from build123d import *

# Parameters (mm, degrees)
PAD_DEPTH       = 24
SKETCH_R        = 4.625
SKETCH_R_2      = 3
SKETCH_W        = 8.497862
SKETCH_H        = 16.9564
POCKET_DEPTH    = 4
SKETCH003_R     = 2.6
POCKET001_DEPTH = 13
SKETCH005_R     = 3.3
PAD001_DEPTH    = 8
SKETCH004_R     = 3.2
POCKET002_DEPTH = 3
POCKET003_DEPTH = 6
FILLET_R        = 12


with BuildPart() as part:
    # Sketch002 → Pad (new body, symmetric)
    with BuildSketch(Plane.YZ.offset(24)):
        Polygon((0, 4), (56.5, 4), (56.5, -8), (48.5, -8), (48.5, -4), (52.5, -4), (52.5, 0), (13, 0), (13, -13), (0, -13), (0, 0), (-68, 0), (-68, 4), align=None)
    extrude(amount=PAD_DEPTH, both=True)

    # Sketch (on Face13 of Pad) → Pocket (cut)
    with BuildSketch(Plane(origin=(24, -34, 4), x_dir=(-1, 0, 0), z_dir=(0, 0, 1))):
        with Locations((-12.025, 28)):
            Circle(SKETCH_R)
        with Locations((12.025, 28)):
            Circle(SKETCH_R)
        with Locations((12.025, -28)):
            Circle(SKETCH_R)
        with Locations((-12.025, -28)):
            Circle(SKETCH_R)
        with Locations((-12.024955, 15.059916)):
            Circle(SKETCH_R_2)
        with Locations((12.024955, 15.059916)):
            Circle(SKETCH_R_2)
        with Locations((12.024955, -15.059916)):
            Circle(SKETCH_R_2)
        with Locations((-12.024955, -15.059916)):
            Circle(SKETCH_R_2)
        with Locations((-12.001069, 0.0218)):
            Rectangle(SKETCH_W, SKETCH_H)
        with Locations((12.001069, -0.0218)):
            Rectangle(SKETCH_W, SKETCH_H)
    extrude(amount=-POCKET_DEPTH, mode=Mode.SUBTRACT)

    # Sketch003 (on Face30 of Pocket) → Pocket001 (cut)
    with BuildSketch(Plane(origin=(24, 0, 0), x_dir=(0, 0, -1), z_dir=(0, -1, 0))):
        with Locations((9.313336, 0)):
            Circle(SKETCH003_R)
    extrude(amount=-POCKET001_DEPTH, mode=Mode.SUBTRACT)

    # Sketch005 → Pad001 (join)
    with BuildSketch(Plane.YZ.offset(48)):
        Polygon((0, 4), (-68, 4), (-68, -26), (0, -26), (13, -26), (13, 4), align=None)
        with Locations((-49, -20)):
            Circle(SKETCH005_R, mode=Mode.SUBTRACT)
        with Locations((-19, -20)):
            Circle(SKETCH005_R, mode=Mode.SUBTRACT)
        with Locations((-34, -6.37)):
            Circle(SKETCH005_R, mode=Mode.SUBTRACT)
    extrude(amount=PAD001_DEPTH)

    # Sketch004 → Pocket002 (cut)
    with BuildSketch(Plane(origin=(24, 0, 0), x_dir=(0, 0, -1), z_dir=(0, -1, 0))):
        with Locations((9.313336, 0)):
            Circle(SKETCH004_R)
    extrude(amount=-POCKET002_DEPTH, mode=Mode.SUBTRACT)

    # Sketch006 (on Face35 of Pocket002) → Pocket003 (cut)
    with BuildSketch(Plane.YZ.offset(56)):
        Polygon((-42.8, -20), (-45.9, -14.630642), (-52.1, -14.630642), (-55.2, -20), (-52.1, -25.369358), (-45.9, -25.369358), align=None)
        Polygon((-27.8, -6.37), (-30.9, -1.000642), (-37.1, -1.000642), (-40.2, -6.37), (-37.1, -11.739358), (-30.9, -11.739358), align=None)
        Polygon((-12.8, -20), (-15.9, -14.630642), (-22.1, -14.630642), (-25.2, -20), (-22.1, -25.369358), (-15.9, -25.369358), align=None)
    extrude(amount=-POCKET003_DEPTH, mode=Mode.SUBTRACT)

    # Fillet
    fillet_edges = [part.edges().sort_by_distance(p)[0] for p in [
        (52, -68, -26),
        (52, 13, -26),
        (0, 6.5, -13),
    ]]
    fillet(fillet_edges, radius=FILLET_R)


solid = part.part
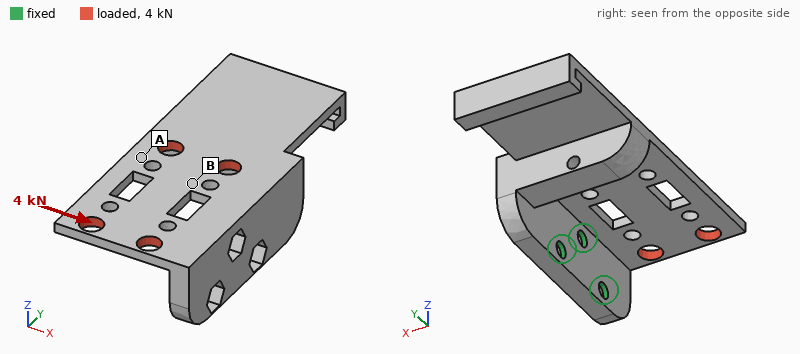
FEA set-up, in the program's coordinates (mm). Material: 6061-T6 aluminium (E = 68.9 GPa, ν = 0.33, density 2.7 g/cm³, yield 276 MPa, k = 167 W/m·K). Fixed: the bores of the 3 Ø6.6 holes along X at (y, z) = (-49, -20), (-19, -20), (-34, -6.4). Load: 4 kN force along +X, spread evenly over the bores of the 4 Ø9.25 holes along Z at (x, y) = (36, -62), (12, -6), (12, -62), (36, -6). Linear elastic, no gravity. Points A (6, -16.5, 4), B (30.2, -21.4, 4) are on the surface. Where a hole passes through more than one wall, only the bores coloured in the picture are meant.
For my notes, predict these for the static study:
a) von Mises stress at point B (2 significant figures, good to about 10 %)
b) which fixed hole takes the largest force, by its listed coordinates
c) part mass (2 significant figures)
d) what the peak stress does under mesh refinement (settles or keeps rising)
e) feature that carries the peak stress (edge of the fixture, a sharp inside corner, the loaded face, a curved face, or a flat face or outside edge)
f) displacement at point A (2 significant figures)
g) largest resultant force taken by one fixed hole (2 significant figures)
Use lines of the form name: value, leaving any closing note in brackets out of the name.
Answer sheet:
von Mises stress at point B: 38 MPa
which fixed hole takes the largest force, by its listed coordinates: (-34, -6.4)
part mass: 130 g
what the peak stress does under mesh refinement: keeps rising
feature that carries the peak stress: edge of the fixture
displacement at point A: 0.19 mm
largest resultant force taken by one fixed hole: 5.0 kN
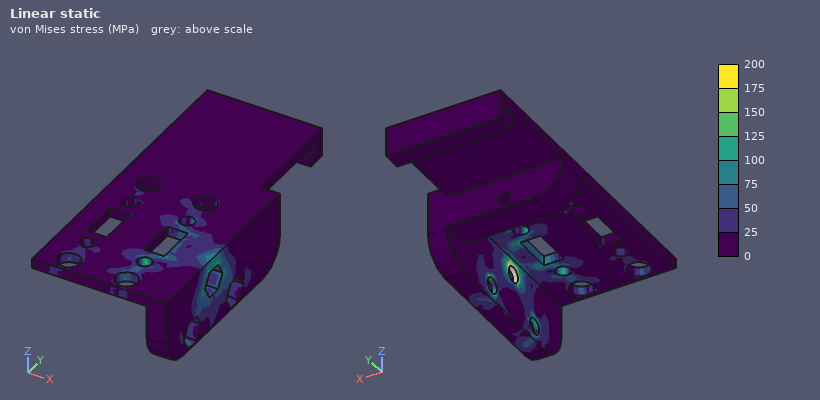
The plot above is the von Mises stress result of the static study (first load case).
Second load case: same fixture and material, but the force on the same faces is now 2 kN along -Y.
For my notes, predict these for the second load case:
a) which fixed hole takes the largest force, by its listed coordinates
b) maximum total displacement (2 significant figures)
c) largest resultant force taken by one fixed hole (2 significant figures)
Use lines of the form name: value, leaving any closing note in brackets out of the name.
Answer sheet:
which fixed hole takes the largest force, by its listed coordinates: (-34, -6.4)
maximum total displacement: 0.52 mm
largest resultant force taken by one fixed hole: 3.1 kN
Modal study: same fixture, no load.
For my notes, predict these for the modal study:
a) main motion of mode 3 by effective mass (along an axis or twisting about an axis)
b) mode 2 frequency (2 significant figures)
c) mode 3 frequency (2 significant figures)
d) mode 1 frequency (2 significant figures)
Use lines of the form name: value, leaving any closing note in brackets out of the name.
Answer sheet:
main motion of mode 3 by effective mass: along Z
mode 2 frequency: 1100 Hz
mode 3 frequency: 1500 Hz
mode 1 frequency: 830 Hz
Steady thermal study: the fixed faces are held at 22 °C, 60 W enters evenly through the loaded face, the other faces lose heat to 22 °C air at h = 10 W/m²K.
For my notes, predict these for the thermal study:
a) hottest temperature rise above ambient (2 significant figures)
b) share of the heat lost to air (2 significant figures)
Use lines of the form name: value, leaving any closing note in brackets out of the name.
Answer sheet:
hottest temperature rise above ambient: 68 K
share of the heat lost to air: 9.6 %
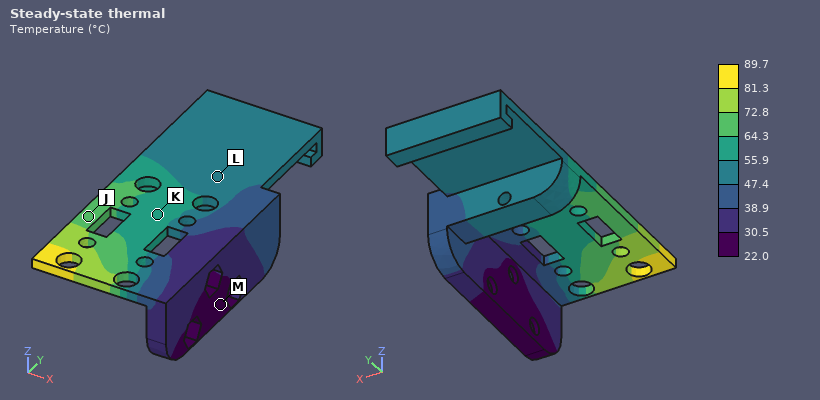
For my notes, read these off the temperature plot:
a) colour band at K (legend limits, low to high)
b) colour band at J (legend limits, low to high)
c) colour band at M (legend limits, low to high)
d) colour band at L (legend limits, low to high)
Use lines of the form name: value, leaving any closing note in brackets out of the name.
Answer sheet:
colour band at K: 55.9 to 64.3 °C
colour band at J: 64.3 to 72.8 °C
colour band at M: 22.0 to 30.5 °C
colour band at L: 47.4 to 55.9 °C
